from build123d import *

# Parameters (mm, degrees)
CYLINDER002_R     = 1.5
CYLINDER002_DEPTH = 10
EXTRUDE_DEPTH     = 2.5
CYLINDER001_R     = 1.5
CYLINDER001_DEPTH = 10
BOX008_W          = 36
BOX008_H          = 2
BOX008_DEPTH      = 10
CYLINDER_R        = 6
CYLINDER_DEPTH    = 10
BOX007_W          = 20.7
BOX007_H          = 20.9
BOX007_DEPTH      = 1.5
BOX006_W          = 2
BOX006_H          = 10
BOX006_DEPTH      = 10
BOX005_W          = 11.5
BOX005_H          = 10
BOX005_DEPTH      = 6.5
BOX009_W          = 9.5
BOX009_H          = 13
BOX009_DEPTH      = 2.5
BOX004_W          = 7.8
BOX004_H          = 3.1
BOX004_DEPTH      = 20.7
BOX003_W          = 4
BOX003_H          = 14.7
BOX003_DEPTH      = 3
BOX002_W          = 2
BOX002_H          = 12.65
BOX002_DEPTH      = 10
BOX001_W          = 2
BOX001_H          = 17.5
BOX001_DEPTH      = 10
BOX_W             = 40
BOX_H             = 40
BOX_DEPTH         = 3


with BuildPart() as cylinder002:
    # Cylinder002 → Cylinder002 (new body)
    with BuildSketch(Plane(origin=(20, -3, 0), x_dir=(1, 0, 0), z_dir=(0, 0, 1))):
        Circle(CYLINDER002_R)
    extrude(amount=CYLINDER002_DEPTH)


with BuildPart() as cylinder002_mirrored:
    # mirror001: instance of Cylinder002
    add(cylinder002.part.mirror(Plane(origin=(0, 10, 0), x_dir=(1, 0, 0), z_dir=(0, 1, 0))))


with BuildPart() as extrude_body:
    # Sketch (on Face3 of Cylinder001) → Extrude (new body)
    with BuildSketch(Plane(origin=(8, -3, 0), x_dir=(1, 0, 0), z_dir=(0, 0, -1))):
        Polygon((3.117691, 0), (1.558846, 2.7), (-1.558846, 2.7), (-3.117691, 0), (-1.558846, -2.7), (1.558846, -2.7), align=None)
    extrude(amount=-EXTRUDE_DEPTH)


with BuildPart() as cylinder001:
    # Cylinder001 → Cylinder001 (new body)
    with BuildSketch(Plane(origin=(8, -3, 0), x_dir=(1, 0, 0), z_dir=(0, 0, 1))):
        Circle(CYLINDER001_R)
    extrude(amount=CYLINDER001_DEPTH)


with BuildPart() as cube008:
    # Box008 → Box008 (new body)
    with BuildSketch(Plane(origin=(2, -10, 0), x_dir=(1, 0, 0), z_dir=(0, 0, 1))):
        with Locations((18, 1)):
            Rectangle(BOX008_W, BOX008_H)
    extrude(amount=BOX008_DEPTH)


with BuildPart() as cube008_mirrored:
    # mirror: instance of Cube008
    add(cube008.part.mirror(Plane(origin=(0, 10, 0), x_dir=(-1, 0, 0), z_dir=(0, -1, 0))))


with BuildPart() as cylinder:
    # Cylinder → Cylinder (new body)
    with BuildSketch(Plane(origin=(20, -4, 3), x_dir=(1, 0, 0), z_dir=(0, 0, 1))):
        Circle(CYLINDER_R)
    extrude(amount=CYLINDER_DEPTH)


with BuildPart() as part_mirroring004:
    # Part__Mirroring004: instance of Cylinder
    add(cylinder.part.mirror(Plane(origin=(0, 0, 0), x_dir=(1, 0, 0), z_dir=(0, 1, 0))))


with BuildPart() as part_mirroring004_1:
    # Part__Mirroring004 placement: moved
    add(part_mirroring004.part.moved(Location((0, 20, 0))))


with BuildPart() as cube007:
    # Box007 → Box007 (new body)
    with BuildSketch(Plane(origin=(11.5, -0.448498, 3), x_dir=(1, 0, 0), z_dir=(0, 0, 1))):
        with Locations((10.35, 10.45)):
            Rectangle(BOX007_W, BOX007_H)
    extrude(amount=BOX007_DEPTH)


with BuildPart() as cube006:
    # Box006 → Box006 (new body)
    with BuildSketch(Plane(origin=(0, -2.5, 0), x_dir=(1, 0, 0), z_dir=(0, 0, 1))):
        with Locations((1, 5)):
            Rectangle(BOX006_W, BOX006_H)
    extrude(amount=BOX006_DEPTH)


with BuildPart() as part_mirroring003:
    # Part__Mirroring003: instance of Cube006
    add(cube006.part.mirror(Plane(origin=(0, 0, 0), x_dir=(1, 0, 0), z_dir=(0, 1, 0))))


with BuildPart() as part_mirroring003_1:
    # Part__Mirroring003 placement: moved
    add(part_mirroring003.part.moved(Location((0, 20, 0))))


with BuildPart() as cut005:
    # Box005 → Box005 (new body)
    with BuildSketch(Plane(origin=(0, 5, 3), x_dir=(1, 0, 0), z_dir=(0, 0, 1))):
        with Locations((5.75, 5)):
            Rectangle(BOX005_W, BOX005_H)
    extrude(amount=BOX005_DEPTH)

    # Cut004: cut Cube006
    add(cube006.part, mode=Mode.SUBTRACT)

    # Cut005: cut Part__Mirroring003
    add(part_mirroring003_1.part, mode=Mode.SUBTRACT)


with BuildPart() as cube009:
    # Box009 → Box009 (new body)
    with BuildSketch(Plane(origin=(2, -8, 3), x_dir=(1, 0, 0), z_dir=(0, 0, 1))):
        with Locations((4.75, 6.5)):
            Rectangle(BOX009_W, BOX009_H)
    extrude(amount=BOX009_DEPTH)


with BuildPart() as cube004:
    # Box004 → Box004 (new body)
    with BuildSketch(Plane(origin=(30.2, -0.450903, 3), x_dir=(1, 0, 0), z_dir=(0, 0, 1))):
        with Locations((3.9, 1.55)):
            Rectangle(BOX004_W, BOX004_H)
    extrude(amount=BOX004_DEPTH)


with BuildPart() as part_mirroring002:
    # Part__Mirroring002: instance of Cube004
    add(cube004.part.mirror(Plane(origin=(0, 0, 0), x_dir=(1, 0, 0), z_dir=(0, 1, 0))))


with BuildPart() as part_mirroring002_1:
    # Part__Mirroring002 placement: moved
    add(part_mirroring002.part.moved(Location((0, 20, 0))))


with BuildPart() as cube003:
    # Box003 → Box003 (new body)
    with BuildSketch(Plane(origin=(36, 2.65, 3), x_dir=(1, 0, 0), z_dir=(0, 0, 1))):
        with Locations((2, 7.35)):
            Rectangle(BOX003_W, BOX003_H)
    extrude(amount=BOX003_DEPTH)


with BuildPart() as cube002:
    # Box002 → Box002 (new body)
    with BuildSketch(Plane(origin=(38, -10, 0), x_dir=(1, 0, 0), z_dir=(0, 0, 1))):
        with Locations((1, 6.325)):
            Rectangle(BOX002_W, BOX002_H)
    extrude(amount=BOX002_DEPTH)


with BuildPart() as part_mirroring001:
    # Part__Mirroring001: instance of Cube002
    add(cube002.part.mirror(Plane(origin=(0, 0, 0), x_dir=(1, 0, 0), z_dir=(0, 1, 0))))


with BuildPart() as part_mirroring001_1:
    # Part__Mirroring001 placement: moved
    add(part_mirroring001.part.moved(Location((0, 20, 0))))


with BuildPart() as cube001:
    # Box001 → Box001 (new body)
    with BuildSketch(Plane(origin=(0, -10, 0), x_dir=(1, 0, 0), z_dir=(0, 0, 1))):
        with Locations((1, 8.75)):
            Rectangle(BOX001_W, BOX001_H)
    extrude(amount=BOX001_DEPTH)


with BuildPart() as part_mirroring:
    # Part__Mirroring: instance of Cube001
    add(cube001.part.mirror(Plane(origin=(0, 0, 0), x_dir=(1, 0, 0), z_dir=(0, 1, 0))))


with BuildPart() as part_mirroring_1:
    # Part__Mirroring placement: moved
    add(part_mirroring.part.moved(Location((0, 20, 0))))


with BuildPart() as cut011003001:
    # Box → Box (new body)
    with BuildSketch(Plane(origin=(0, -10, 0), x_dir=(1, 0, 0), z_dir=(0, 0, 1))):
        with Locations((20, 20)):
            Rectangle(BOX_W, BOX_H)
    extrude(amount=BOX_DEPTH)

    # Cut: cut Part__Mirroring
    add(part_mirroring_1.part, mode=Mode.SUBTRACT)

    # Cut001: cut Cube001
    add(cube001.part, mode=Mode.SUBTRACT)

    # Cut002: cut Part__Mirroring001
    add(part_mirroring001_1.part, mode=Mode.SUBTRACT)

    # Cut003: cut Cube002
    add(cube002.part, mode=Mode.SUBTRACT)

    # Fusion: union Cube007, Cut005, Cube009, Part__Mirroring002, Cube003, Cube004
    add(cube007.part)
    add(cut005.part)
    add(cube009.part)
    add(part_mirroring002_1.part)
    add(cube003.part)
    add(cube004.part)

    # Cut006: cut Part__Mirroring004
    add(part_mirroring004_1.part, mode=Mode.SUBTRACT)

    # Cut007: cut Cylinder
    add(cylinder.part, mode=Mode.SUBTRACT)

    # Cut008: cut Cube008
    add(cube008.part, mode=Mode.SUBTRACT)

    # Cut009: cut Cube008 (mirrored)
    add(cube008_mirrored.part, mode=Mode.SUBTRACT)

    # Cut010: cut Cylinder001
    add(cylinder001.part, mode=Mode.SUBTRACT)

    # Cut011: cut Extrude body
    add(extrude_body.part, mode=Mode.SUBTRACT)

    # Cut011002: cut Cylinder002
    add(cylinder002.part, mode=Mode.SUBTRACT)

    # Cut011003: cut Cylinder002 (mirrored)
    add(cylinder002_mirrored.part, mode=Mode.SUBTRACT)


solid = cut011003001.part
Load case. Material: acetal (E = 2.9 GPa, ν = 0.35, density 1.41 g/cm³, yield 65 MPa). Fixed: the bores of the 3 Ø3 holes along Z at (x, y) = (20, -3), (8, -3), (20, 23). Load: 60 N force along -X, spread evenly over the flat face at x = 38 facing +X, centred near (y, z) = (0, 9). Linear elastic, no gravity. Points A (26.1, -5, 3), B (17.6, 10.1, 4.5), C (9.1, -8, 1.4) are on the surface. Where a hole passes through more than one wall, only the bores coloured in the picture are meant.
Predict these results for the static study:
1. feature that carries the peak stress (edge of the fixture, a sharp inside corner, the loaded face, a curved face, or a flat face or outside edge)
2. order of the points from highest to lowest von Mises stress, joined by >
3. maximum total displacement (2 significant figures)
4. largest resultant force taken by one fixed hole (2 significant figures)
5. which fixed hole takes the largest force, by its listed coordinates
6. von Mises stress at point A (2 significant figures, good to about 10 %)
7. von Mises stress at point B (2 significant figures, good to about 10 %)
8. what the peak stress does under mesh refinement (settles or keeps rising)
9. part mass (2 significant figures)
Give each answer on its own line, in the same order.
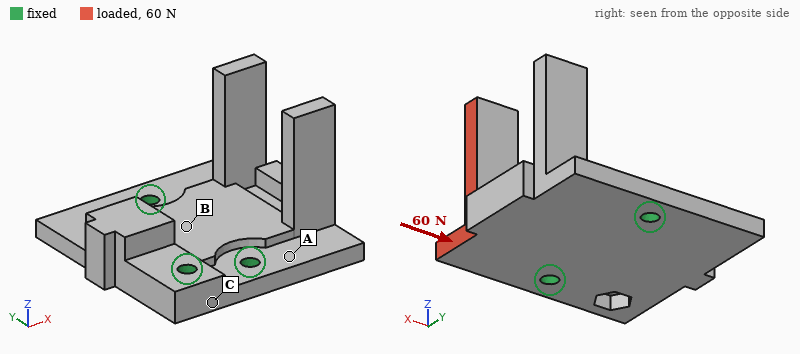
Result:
a sharp inside corner
A > B > C
0.63 mm
38 N
(20, -3)
7.4 MPa
3.0 MPa
keeps rising
9.3 g
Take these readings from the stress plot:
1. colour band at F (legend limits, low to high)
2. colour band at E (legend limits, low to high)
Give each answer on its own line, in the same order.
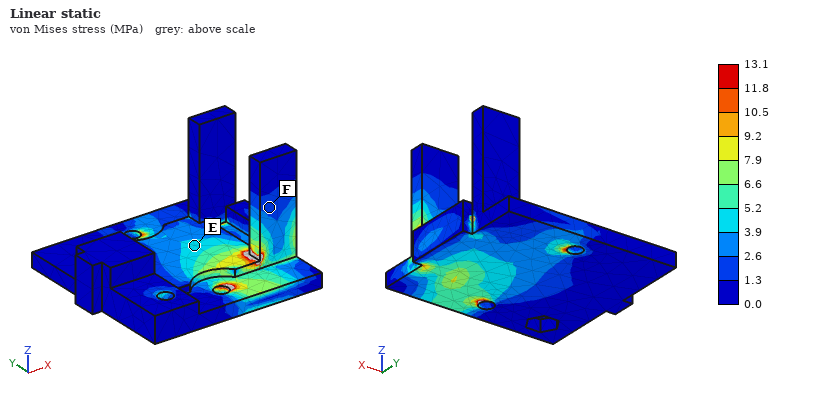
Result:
1.3 to 2.6 MPa
3.9 to 5.2 MPa
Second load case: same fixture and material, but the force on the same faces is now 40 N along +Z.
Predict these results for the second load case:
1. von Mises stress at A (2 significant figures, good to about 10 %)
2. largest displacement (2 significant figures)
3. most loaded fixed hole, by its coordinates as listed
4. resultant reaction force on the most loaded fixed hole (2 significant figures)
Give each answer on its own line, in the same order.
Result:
7.5 MPa
0.59 mm
(20, -3)
59 N
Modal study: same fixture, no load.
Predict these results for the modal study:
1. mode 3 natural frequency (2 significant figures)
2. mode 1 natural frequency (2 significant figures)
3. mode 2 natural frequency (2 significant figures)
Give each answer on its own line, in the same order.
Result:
1400 Hz
1200 Hz
1400 Hz
